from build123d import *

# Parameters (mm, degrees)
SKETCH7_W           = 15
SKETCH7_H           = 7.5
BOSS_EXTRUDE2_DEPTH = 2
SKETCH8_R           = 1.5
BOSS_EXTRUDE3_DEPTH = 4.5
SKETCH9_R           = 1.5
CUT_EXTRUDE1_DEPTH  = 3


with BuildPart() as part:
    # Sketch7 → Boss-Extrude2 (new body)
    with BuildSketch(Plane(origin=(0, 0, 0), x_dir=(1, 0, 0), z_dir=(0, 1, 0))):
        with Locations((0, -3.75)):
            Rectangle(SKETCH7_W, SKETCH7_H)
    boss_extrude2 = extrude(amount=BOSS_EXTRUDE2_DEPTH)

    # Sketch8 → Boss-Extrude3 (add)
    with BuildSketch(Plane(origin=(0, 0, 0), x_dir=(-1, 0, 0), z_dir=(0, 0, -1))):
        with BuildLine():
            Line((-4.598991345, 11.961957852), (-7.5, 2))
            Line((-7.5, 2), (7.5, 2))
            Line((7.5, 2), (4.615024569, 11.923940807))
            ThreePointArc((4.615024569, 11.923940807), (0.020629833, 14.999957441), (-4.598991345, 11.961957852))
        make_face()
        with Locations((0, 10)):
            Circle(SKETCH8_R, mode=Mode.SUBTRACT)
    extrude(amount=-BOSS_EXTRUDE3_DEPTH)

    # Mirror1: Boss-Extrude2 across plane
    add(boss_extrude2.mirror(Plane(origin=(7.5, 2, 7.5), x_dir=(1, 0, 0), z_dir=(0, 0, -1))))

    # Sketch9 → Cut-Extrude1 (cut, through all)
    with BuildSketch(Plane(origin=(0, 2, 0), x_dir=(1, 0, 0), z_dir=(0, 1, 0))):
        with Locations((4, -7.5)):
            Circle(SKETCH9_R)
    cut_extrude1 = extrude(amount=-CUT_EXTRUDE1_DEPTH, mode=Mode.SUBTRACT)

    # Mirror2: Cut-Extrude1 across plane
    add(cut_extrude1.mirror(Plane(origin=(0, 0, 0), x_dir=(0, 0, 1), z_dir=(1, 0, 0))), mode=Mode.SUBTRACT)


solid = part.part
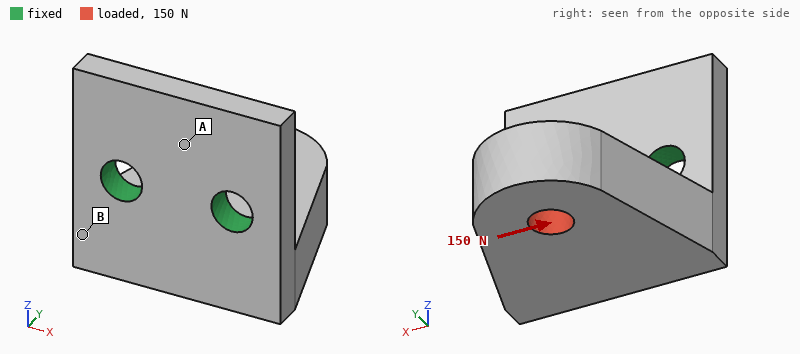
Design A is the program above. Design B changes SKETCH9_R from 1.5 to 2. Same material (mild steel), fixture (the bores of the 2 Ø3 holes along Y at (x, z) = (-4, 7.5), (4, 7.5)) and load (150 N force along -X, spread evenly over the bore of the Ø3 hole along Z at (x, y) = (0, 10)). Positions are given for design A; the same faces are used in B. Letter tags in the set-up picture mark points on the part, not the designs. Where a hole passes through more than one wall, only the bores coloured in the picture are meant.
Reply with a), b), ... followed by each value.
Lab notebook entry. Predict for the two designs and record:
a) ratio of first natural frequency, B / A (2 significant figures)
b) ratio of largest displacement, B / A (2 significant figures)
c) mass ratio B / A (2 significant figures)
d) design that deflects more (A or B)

a) 1.1
b) 0.76
c) 0.98
d) A
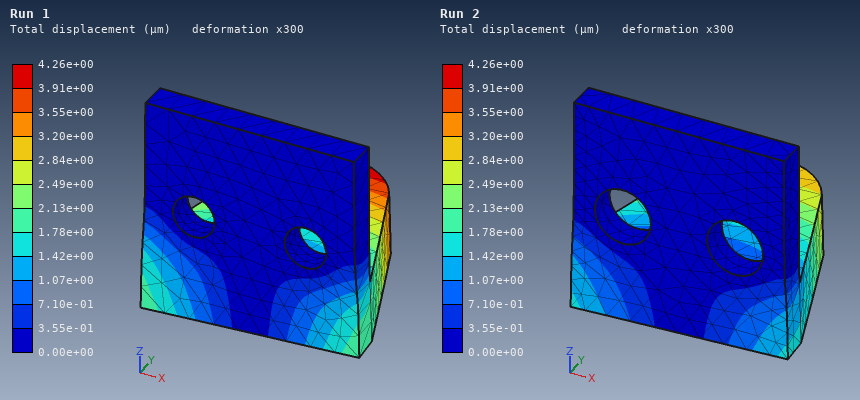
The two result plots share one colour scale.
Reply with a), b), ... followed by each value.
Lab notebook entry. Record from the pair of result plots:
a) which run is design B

a) Run 2
